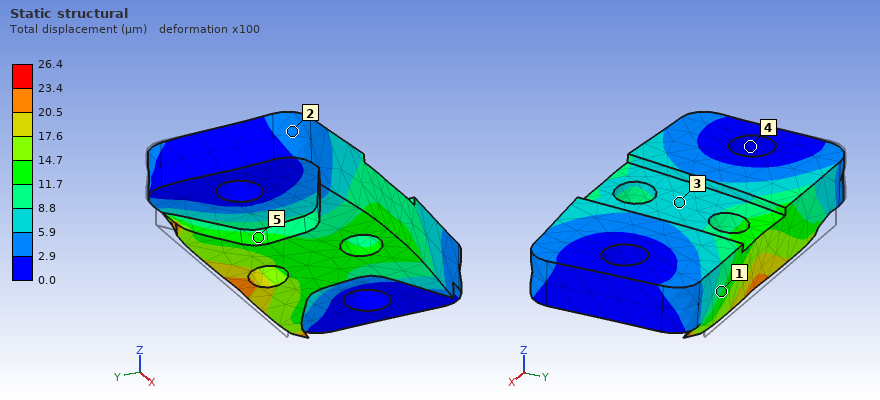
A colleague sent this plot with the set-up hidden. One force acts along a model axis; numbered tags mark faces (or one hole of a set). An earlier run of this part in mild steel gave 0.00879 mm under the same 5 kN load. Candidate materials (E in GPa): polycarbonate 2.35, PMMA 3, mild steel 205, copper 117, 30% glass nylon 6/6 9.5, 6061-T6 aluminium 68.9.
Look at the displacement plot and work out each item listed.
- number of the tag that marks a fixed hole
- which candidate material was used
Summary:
4
6061-T6 aluminium
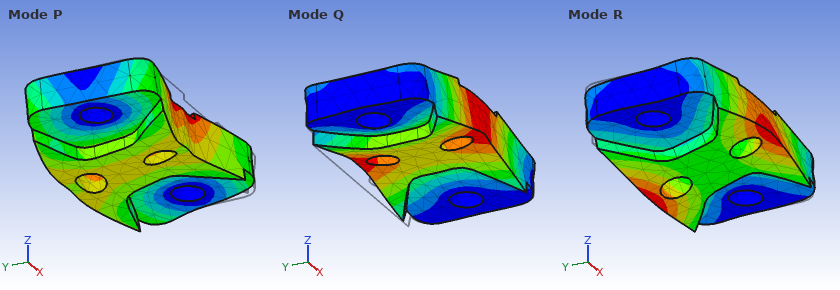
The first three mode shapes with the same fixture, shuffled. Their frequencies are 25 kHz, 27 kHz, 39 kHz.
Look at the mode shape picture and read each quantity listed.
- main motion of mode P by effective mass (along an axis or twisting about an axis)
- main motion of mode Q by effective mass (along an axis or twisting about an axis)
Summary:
along Y
along Z
